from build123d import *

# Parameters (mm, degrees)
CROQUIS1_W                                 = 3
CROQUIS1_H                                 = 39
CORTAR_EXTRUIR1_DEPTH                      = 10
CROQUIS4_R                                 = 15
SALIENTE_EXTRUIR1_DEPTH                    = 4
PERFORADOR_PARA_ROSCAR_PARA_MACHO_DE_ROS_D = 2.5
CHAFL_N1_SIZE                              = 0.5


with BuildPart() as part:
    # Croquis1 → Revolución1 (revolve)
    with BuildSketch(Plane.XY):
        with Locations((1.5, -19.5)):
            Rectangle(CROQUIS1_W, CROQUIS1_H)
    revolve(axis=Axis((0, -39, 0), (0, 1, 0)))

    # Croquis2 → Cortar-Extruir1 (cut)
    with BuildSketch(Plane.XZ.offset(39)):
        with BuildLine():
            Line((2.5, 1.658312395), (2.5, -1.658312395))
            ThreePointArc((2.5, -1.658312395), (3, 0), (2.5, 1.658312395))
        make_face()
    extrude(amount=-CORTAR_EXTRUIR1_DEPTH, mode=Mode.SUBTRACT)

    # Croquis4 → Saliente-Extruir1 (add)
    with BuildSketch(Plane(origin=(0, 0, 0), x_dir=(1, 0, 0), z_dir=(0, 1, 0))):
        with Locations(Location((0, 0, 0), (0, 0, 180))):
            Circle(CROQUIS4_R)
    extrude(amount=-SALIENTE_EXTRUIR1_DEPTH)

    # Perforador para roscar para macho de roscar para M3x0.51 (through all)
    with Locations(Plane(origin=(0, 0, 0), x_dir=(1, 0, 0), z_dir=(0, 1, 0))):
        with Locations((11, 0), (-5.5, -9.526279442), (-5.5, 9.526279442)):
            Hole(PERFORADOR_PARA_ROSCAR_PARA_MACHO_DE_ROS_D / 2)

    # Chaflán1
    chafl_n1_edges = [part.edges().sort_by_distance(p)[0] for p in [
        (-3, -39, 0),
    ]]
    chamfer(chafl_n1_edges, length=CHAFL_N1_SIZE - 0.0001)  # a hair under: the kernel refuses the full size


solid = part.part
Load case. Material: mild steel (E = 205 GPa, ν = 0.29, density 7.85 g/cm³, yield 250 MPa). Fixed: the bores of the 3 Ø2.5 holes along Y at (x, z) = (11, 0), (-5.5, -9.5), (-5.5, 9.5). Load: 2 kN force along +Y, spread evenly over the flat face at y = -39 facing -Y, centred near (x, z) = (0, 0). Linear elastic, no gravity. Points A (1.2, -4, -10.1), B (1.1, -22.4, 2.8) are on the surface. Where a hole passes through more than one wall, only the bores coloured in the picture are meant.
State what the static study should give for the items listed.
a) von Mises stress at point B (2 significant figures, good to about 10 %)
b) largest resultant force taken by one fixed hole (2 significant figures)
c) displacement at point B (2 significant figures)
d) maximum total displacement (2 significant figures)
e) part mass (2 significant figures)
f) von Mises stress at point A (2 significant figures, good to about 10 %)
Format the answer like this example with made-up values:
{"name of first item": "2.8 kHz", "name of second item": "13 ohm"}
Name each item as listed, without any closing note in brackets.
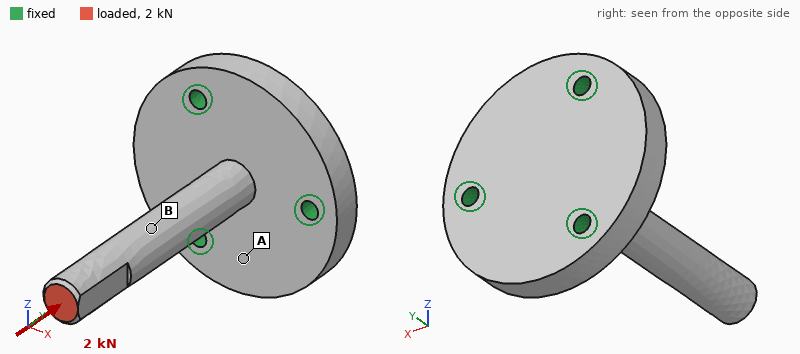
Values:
{"von Mises stress at point B": "71 MPa", "largest resultant force taken by one fixed hole": "670 N", "displacement at point B": "12 µm", "maximum total displacement": "19 µm", "part mass": "29 g", "von Mises stress at point A": "22 MPa"}
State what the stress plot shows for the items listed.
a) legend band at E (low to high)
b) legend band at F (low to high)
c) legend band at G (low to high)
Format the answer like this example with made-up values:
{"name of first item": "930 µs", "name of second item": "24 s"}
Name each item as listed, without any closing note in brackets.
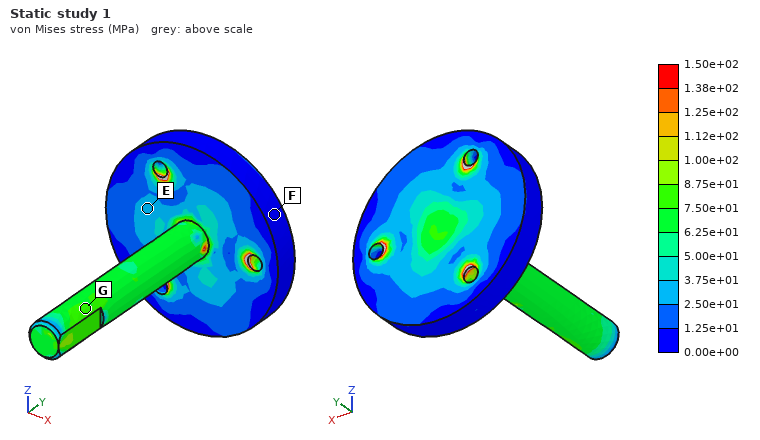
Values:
{"legend band at E": "2.50e+01 to 3.75e+01 MPa", "legend band at F": "0.00e+00 to 1.25e+01 MPa", "legend band at G": "7.50e+01 to 8.75e+01 MPa"}
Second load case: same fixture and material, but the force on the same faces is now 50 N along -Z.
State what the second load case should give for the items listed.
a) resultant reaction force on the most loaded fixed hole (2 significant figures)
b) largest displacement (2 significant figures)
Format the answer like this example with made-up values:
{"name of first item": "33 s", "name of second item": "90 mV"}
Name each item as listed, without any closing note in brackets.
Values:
{"resultant reaction force on the most loaded fixed hole": "100 N", "largest displacement": "66 µm"}
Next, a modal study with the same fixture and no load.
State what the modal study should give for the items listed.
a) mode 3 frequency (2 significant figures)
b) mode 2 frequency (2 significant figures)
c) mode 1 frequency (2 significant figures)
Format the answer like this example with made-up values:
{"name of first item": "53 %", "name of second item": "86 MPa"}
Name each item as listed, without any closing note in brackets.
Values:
{"mode 3 frequency": "18 kHz", "mode 2 frequency": "3100 Hz", "mode 1 frequency": "3100 Hz"}
